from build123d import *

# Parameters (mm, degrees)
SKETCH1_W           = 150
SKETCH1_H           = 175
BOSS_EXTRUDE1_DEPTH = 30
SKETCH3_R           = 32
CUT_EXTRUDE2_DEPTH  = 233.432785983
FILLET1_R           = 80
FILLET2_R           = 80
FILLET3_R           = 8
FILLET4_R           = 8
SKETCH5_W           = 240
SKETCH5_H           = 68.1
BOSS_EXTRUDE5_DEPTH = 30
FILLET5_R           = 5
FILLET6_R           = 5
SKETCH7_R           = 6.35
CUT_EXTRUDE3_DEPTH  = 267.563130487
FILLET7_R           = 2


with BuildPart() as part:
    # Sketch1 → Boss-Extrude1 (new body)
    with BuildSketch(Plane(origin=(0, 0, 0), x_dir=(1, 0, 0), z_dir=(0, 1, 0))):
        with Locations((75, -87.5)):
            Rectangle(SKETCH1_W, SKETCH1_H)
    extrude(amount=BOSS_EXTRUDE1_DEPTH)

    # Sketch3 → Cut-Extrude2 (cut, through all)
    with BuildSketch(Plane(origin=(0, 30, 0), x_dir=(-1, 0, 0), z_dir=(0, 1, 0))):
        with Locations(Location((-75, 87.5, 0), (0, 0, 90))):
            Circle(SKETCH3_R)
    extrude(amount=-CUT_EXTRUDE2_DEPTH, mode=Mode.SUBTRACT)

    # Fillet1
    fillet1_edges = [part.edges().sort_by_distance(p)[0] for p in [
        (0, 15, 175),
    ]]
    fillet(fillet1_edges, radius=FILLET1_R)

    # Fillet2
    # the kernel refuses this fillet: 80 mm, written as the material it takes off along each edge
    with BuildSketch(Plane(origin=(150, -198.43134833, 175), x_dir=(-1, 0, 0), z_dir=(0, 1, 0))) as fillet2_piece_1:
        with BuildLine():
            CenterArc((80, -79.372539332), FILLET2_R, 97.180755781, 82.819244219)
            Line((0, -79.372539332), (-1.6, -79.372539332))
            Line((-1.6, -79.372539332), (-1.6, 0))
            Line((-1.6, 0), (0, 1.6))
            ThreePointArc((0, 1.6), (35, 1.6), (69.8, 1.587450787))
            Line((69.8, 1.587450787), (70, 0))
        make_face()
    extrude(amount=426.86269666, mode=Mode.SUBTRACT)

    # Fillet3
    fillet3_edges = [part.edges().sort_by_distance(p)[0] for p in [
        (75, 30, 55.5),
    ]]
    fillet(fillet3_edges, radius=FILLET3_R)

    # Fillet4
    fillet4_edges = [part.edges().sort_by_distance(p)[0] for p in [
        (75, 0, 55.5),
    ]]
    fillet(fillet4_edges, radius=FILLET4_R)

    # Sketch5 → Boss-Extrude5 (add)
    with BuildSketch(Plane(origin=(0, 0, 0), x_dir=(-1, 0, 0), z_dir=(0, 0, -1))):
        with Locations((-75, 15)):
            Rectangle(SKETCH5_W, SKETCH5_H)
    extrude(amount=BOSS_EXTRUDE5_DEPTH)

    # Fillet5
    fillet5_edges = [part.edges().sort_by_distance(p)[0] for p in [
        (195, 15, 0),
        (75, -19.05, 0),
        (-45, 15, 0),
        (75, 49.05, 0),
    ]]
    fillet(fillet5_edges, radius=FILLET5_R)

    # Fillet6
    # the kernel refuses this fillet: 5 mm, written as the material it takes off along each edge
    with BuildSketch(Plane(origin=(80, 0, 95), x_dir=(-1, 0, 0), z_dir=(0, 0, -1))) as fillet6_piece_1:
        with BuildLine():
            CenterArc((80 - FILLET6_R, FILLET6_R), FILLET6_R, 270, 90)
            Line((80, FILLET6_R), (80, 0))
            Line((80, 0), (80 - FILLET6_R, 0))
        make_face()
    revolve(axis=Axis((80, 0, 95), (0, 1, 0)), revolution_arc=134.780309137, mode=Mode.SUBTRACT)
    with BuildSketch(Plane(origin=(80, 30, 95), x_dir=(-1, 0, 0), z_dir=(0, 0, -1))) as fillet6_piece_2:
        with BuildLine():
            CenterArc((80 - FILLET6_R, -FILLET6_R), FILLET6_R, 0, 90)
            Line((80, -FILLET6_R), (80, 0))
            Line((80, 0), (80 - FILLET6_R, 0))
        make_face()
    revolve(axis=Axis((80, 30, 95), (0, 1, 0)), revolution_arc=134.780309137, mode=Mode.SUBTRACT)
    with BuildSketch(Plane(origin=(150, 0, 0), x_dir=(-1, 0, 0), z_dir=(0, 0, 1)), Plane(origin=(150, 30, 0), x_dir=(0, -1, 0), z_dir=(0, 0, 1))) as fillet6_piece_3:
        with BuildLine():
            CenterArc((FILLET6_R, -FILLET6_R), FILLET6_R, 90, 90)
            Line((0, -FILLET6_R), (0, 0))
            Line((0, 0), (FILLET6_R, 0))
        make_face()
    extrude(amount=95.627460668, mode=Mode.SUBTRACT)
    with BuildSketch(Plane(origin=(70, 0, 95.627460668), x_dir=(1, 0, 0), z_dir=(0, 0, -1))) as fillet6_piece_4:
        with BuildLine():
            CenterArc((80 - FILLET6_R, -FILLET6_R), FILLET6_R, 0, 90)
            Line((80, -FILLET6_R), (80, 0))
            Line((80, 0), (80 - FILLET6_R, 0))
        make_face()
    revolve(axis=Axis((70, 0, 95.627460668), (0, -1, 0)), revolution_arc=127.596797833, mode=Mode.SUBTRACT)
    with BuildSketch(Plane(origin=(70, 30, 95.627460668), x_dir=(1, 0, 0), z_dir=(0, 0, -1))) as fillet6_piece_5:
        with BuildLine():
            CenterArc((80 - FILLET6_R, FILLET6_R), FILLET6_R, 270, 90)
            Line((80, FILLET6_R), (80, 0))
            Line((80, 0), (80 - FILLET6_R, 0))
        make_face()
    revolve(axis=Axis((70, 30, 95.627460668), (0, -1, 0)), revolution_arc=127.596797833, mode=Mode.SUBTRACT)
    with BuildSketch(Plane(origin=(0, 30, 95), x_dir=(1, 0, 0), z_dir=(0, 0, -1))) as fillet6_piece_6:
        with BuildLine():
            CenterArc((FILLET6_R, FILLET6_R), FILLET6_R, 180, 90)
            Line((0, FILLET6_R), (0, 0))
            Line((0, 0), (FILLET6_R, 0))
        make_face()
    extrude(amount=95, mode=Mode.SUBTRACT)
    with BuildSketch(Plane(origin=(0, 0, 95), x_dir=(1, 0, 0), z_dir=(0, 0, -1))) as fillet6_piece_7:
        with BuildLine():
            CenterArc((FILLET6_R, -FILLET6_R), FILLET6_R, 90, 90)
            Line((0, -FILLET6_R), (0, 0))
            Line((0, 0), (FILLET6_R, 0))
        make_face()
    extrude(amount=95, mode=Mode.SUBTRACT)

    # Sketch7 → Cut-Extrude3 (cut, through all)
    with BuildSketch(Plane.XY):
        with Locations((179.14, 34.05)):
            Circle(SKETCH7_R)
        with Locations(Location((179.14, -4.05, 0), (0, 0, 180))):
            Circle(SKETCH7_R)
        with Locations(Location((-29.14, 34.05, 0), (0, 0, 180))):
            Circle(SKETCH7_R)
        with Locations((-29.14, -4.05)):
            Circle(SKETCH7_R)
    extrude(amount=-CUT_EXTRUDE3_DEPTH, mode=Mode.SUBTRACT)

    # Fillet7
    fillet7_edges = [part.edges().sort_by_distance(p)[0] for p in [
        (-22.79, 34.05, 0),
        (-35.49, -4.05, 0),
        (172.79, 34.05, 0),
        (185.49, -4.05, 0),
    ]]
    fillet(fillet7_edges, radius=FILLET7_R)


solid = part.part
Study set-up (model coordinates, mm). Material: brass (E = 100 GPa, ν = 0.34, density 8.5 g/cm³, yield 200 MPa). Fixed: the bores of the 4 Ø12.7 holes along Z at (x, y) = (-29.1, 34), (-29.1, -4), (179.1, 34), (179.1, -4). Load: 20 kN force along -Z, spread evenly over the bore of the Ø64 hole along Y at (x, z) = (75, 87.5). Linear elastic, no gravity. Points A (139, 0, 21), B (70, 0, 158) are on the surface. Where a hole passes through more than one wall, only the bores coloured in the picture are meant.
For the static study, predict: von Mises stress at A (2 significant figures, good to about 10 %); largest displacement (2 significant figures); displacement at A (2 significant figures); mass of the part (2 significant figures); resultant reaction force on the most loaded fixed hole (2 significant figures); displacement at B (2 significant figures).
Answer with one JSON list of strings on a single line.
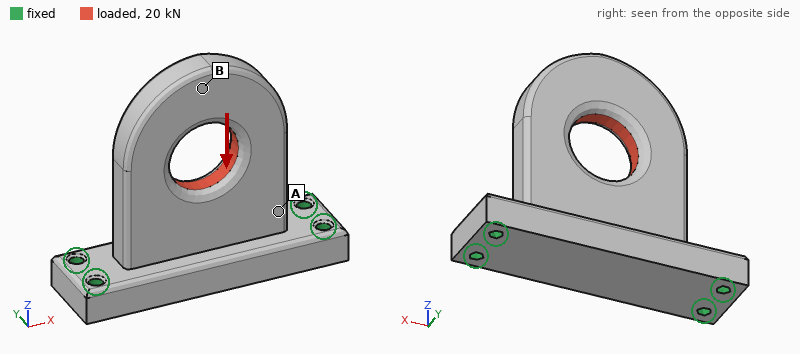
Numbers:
["10 MPa", "22 µm", "14 µm", "9.1 kg", "5.5 kN", "21 µm"]
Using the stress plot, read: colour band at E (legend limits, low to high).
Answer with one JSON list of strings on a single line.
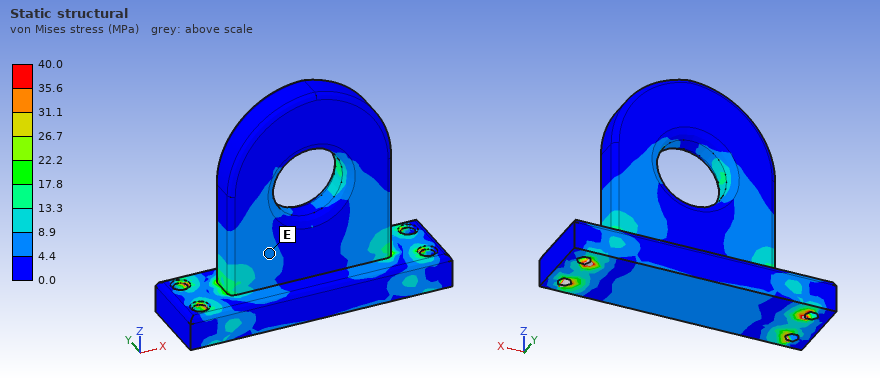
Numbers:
["4.4 to 8.9 MPa"]
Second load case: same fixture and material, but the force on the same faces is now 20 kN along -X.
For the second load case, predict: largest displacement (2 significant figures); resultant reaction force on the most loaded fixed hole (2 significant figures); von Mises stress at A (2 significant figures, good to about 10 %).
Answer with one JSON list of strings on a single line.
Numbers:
["70 µm", "8.0 kN", "15 MPa"]
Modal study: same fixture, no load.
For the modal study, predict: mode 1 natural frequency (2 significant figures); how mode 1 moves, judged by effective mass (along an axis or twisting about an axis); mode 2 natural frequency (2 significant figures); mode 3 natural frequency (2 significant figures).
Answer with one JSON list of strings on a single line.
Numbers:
["430 Hz", "along Y", "1400 Hz", "1400 Hz"]
